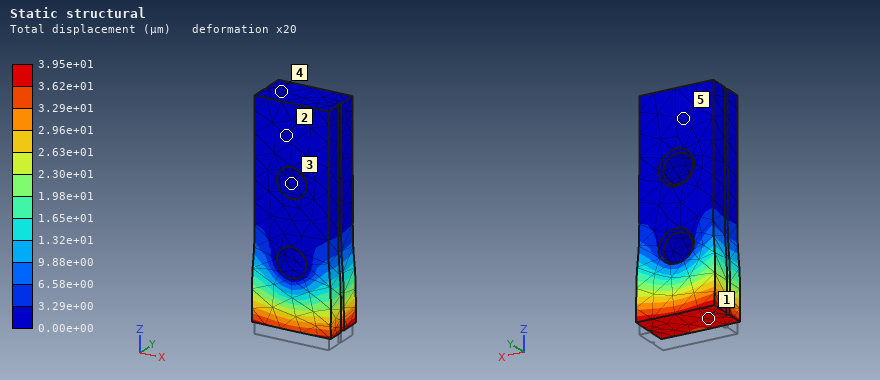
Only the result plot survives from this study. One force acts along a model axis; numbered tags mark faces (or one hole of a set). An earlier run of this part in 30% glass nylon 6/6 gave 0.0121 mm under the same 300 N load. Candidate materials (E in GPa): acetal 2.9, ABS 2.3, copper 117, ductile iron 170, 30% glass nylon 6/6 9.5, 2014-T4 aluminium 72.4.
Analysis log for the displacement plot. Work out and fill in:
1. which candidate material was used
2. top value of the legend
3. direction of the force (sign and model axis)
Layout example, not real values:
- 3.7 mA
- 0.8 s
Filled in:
- acetal
- 3.95e+01 µm
- +Z
